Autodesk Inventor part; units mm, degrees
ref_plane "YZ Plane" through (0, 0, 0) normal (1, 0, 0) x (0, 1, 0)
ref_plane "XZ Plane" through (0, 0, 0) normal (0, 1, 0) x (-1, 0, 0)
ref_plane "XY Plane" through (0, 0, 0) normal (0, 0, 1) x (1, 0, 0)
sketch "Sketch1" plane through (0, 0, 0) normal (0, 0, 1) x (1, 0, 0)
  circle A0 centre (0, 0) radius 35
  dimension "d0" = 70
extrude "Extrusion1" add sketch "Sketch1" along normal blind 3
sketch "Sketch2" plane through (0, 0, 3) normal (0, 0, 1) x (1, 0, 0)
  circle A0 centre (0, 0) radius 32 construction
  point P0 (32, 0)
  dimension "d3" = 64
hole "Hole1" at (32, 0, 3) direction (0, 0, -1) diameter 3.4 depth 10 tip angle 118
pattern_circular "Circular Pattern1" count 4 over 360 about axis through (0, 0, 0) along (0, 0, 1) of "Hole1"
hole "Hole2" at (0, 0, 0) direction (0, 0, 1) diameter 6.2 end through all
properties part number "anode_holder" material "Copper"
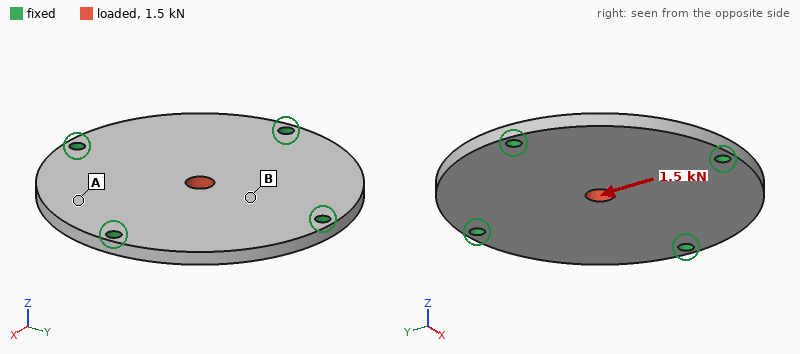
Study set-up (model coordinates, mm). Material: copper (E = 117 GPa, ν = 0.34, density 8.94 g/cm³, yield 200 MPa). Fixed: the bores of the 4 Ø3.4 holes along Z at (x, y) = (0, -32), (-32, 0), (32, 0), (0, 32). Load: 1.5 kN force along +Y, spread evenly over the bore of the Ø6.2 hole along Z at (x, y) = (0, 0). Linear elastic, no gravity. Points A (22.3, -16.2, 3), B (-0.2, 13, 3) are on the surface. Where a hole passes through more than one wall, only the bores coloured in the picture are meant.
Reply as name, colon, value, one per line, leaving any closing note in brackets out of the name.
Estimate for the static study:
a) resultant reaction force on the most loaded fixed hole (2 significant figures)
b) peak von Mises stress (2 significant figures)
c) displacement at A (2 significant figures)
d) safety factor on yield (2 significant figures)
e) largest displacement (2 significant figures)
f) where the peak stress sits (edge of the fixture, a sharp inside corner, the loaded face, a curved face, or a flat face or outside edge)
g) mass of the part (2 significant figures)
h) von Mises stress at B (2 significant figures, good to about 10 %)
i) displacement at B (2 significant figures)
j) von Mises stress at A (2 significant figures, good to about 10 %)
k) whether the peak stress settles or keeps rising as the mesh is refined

resultant reaction force on the most loaded fixed hole: 490 N
peak von Mises stress: 44 MPa
displacement at A: 1.3 µm
safety factor on yield: 4.6
largest displacement: 3.8 µm
where the peak stress sits: the loaded face
mass of the part: 100 g
von Mises stress at B: 14 MPa
displacement at B: 2.2 µm
von Mises stress at A: 3.1 MPa
whether the peak stress settles or keeps rising as the mesh is refined: settles
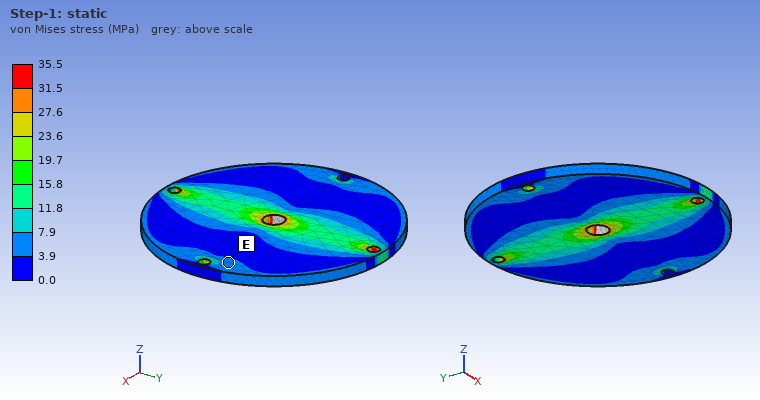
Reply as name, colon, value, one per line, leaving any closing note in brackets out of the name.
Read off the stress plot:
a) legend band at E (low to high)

legend band at E: 3.9 to 7.9 MPa
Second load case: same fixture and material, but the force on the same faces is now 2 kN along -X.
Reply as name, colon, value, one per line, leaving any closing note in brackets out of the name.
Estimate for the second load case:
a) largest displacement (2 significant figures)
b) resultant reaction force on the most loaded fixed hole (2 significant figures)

largest displacement: 5.1 µm
resultant reaction force on the most loaded fixed hole: 650 N
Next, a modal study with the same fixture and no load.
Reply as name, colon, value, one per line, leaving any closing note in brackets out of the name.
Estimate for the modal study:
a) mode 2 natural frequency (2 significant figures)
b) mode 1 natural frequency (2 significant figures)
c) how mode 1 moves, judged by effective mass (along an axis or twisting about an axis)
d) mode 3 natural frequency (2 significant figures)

mode 2 natural frequency: 4600 Hz
mode 1 natural frequency: 3800 Hz
how mode 1 moves, judged by effective mass: along Z
mode 3 natural frequency: 4900 Hz
